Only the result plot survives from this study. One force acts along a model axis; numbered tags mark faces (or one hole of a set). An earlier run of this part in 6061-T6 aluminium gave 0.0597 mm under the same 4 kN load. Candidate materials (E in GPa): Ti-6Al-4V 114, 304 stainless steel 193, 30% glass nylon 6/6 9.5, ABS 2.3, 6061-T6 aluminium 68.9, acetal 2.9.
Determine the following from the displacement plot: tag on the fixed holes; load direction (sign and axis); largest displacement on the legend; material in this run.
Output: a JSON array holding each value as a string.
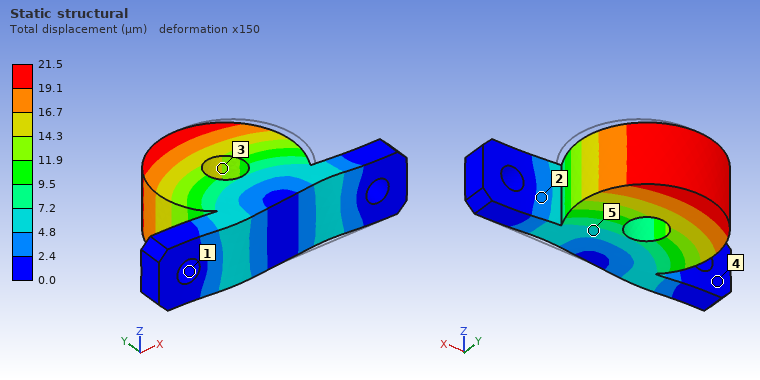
["1", "-X", "21.5 µm", "304 stainless steel"]
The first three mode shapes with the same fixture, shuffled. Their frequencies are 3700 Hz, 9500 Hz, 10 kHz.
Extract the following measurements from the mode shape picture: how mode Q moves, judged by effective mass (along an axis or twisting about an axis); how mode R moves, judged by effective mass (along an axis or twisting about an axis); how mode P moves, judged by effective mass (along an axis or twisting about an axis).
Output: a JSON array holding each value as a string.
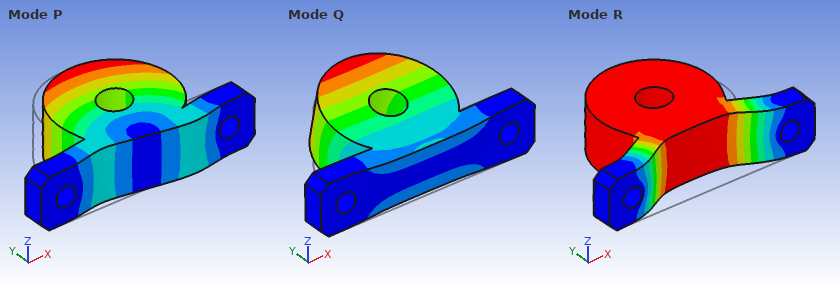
["along Z", "along Y", "along X"]
